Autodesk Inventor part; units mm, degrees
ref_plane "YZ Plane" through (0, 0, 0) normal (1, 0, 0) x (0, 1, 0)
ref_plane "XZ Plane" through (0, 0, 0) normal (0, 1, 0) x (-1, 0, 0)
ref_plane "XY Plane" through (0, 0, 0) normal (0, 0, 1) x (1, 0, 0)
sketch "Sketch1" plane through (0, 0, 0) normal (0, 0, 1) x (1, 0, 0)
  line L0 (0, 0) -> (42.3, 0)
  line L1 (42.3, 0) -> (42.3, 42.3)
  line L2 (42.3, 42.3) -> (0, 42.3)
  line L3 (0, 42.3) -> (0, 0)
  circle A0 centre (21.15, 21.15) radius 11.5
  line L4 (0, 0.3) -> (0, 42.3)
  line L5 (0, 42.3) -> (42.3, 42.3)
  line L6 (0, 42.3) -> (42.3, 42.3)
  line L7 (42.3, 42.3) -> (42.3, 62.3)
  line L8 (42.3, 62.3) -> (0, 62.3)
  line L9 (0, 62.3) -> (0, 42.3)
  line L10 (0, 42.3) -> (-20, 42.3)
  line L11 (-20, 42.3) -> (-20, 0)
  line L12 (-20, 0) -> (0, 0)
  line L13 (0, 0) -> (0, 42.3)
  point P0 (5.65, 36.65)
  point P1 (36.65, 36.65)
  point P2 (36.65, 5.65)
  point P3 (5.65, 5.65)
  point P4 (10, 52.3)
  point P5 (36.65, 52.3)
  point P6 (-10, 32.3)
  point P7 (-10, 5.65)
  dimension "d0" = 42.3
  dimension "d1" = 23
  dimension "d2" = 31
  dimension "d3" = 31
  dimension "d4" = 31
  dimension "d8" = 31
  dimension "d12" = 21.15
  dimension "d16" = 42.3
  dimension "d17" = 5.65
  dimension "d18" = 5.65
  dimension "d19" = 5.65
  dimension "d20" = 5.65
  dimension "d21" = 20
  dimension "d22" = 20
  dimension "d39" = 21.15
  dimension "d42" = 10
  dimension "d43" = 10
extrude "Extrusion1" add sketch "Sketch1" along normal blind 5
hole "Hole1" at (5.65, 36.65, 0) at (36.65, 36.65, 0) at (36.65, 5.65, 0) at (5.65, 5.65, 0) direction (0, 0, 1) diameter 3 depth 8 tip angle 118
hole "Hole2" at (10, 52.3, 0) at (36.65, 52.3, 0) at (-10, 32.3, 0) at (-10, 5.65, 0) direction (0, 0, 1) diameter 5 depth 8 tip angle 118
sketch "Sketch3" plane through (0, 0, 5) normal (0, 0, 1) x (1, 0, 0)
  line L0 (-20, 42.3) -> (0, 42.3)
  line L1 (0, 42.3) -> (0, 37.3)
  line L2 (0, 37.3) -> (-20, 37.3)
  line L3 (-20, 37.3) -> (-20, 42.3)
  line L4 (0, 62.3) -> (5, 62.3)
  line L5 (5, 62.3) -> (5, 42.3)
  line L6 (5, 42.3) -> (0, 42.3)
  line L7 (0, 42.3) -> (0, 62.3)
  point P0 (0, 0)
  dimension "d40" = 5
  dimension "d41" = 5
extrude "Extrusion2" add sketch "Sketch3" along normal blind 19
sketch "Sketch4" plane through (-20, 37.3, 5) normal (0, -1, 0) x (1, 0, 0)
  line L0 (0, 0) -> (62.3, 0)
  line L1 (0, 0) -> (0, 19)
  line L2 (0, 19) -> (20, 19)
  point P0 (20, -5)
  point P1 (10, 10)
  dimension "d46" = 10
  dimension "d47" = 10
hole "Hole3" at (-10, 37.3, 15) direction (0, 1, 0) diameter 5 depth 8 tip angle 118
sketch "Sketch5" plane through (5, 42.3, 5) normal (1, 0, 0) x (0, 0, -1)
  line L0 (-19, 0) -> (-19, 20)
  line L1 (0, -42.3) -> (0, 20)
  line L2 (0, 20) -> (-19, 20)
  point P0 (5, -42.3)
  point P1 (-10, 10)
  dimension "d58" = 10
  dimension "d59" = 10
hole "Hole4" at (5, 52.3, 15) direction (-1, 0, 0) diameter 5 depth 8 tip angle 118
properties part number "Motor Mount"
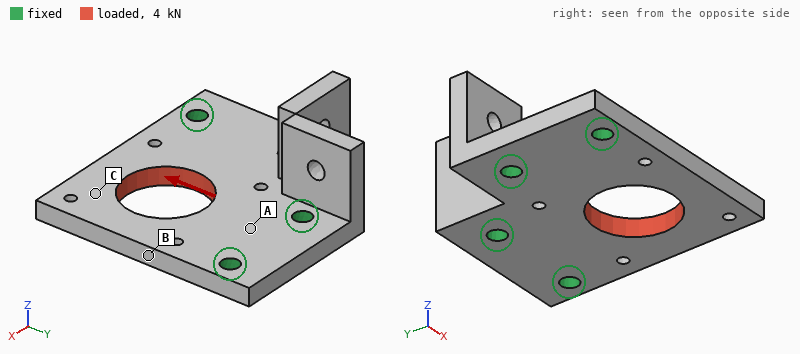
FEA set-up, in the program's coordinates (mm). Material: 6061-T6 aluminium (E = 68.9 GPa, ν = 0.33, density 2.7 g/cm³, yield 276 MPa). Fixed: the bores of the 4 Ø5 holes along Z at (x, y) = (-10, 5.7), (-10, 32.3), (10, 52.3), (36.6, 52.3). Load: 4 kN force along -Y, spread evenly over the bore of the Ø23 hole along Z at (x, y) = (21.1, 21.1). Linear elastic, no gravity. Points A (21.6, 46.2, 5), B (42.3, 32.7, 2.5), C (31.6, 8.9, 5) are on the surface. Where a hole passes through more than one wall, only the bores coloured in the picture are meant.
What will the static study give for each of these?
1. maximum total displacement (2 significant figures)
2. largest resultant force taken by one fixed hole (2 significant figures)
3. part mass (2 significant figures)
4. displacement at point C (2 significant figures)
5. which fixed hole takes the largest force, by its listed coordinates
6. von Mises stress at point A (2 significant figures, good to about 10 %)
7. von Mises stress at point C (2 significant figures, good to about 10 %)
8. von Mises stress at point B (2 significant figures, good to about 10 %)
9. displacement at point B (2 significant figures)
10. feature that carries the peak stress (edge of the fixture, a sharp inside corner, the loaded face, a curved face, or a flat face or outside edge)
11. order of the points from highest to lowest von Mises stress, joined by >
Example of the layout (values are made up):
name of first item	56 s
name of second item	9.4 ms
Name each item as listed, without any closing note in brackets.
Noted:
maximum total displacement	19 µm
largest resultant force taken by one fixed hole	1.7 kN
part mass	50 g
displacement at point C	16 µm
which fixed hole takes the largest force, by its listed coordinates	(36.6, 52.3)
von Mises stress at point A	6.2 MPa
von Mises stress at point C	13 MPa
von Mises stress at point B	25 MPa
displacement at point B	9.1 µm
feature that carries the peak stress	a curved face
order of the points from highest to lowest von Mises stress, joined by >	B > C > A
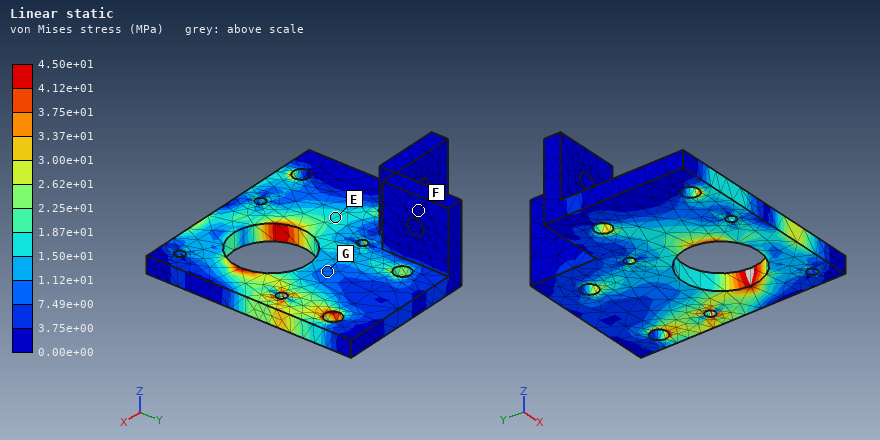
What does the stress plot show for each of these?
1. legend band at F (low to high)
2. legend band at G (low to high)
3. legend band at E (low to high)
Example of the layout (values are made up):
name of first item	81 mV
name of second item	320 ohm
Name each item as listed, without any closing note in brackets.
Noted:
legend band at F	0.00e+00 to 3.75e+00 MPa
legend band at G	7.49e+00 to 1.12e+01 MPa
legend band at E	1.50e+01 to 1.87e+01 MPa
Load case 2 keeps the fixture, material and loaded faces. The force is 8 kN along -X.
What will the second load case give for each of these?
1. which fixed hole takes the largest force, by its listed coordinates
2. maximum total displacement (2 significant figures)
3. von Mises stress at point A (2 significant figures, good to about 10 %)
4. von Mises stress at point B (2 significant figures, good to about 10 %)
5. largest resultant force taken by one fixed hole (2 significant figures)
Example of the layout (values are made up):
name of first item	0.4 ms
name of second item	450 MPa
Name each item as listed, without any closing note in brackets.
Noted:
which fixed hole takes the largest force, by its listed coordinates	(-10, 5.7)
maximum total displacement	38 µm
von Mises stress at point A	26 MPa
von Mises stress at point B	13 MPa
largest resultant force taken by one fixed hole	3.5 kN
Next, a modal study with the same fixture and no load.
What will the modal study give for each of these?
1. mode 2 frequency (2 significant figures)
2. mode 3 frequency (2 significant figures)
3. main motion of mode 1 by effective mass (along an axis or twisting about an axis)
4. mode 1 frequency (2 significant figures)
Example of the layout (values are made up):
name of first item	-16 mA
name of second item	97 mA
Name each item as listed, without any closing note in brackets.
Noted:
mode 2 frequency	8000 Hz
mode 3 frequency	9200 Hz
main motion of mode 1 by effective mass	along Z
mode 1 frequency	2900 Hz
